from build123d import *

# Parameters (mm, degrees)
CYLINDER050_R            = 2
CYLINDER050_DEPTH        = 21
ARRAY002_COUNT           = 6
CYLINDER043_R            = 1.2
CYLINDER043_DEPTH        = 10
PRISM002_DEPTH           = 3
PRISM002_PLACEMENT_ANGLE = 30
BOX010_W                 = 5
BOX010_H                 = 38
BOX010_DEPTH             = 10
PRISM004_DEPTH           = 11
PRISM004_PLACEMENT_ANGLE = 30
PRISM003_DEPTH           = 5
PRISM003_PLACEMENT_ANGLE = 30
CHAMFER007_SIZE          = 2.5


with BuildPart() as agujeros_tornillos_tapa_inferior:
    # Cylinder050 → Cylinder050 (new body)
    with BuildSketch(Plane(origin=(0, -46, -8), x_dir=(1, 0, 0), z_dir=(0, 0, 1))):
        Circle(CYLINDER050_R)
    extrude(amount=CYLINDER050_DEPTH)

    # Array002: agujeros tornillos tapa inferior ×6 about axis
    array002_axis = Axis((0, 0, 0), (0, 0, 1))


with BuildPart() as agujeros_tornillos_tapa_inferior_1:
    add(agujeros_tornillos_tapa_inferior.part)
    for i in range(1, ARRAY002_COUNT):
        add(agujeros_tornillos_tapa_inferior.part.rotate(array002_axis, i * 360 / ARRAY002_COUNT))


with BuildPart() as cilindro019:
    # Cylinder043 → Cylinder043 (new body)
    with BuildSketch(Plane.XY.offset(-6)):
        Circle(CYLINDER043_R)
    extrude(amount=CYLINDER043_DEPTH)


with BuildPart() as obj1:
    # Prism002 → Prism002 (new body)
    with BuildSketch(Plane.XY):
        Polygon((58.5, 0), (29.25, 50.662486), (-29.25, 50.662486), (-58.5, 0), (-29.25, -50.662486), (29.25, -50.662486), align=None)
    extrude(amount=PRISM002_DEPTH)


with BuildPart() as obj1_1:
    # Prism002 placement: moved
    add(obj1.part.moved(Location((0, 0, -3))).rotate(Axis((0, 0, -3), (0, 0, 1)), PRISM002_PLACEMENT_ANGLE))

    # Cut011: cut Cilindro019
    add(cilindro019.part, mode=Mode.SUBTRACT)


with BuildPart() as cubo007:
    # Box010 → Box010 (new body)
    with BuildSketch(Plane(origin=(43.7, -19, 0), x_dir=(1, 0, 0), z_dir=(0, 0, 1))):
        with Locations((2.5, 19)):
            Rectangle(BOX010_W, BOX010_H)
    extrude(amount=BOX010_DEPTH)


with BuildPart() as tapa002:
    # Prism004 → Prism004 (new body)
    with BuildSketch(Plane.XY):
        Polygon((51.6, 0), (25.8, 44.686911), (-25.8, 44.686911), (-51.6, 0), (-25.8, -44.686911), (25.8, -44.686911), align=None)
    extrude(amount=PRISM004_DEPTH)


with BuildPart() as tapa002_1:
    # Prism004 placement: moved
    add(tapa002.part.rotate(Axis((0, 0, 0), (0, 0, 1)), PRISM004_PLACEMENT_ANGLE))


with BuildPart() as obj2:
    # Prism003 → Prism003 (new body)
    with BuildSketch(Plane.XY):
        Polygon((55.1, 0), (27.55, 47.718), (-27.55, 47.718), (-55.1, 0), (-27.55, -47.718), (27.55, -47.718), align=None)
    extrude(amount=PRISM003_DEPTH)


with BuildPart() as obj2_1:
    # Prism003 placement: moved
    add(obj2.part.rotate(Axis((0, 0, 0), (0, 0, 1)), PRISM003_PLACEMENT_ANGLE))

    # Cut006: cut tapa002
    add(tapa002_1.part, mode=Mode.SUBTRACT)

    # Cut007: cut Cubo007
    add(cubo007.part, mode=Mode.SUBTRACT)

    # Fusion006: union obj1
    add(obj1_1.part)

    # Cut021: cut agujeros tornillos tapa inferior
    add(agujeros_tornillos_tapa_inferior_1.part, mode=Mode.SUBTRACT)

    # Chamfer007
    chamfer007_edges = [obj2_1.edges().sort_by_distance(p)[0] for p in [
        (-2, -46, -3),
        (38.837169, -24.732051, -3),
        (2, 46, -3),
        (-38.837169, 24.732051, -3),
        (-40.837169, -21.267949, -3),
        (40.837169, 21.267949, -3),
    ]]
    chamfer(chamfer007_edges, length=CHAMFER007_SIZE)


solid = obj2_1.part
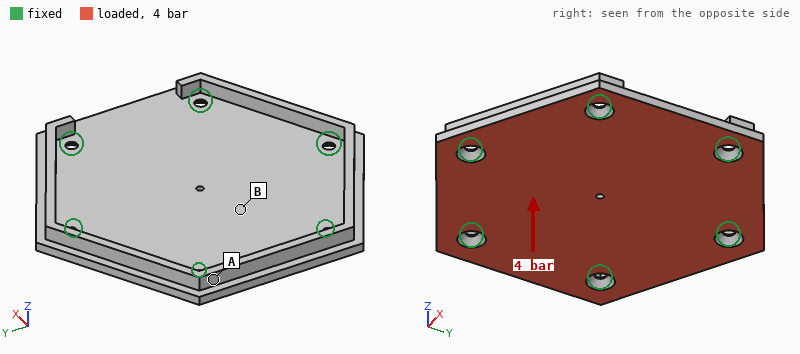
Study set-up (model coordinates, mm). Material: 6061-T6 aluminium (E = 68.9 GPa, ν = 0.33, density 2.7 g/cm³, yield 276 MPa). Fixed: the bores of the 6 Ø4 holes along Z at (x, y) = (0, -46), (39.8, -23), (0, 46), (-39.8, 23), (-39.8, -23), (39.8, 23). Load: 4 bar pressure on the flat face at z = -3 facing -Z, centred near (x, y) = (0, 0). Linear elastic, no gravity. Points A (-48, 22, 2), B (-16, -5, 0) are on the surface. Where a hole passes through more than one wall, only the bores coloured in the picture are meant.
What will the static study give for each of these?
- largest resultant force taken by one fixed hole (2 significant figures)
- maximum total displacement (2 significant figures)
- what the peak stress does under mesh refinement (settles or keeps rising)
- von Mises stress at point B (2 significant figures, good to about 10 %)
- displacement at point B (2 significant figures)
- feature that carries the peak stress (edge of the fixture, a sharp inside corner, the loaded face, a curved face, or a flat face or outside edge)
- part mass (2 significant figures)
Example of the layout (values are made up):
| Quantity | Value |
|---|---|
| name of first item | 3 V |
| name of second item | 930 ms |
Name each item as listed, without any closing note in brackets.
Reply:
| Quantity | Value |
|---|---|
| largest resultant force taken by one fixed hole | 1.2 kN |
| maximum total displacement | 0.29 mm |
| what the peak stress does under mesh refinement | keeps rising |
| von Mises stress at point B | 44 MPa |
| displacement at point B | 0.23 mm |
| feature that carries the peak stress | edge of the fixture |
| part mass | 82 g |
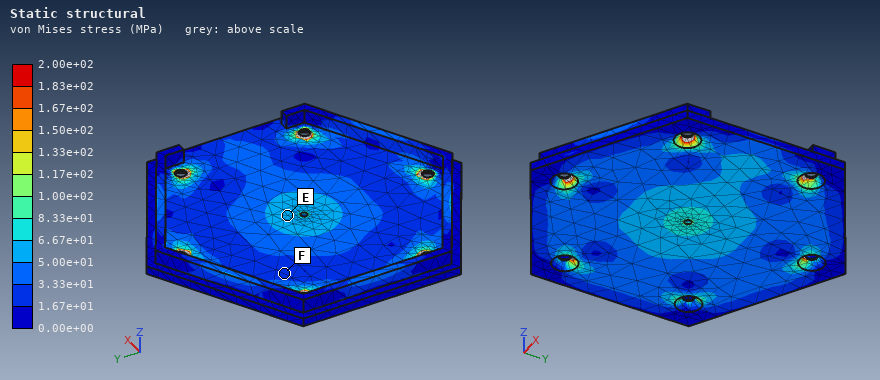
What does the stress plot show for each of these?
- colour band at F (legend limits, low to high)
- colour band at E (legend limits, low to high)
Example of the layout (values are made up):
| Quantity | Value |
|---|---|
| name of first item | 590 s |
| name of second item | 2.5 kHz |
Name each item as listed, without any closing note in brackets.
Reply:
| Quantity | Value |
|---|---|
| colour band at F | 1.67e+01 to 3.33e+01 MPa |
| colour band at E | 5.00e+01 to 6.67e+01 MPa |
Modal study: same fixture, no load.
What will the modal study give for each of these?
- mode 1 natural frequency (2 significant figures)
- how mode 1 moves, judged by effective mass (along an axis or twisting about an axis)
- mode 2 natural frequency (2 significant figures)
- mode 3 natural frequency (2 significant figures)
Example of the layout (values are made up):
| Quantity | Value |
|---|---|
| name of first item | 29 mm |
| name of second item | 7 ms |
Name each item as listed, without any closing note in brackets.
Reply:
| Quantity | Value |
|---|---|
| mode 1 natural frequency | 2500 Hz |
| how mode 1 moves, judged by effective mass | along Z |
| mode 2 natural frequency | 5200 Hz |
| mode 3 natural frequency | 5400 Hz |
